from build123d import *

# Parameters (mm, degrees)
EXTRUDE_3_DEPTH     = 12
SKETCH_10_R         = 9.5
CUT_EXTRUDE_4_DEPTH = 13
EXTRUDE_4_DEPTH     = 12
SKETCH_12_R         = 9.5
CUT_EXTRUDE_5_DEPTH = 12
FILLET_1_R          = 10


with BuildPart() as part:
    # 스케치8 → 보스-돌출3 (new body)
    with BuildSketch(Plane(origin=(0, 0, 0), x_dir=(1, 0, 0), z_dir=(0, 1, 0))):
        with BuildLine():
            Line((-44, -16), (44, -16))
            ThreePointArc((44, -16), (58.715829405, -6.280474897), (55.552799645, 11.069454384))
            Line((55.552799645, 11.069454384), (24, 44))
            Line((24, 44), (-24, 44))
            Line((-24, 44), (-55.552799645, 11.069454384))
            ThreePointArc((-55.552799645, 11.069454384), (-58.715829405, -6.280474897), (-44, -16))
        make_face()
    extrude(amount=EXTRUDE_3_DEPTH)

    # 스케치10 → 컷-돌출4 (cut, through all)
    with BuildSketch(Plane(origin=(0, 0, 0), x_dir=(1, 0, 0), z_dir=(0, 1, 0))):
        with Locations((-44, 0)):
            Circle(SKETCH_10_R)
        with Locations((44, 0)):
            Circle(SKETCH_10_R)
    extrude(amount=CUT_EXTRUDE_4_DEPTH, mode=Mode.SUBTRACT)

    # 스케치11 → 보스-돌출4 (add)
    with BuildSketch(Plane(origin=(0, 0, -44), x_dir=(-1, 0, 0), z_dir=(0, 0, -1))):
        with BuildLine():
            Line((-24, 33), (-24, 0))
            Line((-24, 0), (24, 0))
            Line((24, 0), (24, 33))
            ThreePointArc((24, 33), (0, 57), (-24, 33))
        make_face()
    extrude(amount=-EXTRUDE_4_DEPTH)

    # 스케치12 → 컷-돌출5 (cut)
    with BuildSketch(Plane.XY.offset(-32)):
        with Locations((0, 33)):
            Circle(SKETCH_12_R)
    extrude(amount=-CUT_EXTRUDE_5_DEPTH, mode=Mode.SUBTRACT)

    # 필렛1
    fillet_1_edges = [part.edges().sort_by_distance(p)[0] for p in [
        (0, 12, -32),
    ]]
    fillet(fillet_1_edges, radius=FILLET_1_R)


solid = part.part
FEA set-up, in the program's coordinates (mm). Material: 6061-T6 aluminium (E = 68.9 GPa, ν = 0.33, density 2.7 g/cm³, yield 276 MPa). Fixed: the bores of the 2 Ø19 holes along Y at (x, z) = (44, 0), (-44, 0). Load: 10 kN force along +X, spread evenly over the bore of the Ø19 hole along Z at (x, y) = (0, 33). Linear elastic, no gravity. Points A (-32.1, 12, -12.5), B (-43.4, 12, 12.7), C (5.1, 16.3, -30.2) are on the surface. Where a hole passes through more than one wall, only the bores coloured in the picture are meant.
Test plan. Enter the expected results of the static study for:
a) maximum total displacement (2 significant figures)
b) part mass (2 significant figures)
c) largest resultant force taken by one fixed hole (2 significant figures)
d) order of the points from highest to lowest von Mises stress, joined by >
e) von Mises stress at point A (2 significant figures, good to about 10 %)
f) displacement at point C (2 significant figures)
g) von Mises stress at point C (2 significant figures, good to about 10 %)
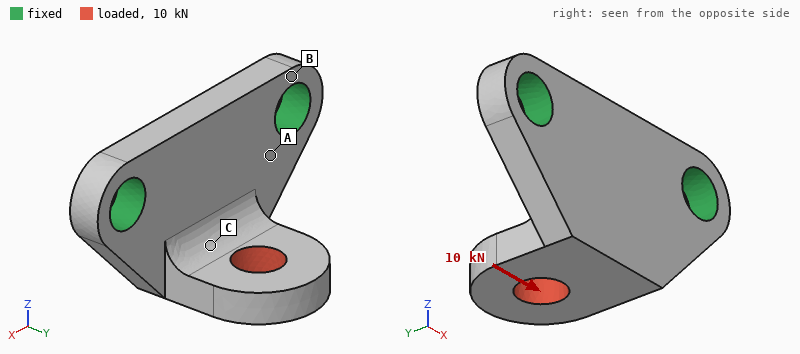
0.20 mm
220 g
7.5 kN
C > A > B
40 MPa
0.043 mm
94 MPa
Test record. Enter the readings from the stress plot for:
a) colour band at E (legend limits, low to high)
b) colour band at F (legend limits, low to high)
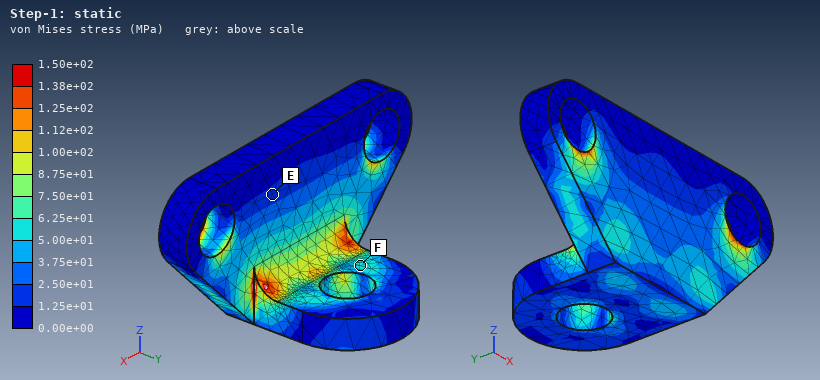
1.25e+01 to 2.50e+01 MPa
5.00e+01 to 6.25e+01 MPa
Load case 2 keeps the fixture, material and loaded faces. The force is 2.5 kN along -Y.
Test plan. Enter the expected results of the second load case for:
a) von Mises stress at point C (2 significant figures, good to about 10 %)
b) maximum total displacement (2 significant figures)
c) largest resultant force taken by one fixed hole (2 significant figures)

8.7 MPa
0.13 mm
1.3 kN
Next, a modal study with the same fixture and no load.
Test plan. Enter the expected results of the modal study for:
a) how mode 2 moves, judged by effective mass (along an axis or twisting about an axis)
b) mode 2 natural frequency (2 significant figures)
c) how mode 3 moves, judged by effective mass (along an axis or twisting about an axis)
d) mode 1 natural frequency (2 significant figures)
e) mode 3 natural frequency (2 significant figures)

along X
5300 Hz
along Y
2500 Hz
5500 Hz
